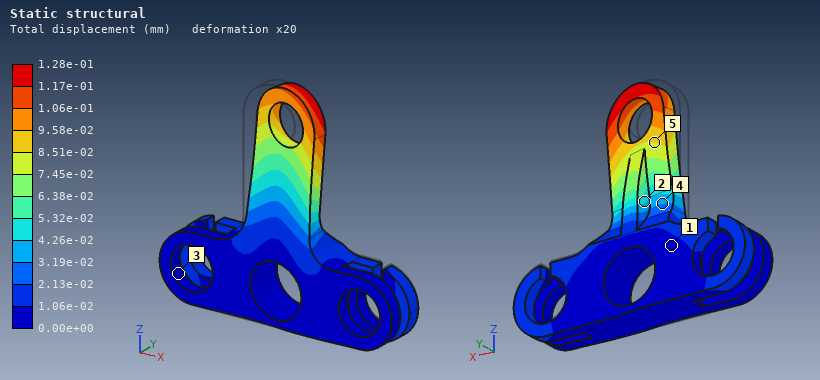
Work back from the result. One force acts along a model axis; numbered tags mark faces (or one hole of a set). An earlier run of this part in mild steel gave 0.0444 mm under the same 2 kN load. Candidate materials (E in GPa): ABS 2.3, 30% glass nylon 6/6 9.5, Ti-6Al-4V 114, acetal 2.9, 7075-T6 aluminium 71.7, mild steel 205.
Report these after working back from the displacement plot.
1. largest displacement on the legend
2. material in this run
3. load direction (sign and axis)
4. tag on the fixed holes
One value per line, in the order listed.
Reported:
1.28e-01 mm
7075-T6 aluminium
+X
3
